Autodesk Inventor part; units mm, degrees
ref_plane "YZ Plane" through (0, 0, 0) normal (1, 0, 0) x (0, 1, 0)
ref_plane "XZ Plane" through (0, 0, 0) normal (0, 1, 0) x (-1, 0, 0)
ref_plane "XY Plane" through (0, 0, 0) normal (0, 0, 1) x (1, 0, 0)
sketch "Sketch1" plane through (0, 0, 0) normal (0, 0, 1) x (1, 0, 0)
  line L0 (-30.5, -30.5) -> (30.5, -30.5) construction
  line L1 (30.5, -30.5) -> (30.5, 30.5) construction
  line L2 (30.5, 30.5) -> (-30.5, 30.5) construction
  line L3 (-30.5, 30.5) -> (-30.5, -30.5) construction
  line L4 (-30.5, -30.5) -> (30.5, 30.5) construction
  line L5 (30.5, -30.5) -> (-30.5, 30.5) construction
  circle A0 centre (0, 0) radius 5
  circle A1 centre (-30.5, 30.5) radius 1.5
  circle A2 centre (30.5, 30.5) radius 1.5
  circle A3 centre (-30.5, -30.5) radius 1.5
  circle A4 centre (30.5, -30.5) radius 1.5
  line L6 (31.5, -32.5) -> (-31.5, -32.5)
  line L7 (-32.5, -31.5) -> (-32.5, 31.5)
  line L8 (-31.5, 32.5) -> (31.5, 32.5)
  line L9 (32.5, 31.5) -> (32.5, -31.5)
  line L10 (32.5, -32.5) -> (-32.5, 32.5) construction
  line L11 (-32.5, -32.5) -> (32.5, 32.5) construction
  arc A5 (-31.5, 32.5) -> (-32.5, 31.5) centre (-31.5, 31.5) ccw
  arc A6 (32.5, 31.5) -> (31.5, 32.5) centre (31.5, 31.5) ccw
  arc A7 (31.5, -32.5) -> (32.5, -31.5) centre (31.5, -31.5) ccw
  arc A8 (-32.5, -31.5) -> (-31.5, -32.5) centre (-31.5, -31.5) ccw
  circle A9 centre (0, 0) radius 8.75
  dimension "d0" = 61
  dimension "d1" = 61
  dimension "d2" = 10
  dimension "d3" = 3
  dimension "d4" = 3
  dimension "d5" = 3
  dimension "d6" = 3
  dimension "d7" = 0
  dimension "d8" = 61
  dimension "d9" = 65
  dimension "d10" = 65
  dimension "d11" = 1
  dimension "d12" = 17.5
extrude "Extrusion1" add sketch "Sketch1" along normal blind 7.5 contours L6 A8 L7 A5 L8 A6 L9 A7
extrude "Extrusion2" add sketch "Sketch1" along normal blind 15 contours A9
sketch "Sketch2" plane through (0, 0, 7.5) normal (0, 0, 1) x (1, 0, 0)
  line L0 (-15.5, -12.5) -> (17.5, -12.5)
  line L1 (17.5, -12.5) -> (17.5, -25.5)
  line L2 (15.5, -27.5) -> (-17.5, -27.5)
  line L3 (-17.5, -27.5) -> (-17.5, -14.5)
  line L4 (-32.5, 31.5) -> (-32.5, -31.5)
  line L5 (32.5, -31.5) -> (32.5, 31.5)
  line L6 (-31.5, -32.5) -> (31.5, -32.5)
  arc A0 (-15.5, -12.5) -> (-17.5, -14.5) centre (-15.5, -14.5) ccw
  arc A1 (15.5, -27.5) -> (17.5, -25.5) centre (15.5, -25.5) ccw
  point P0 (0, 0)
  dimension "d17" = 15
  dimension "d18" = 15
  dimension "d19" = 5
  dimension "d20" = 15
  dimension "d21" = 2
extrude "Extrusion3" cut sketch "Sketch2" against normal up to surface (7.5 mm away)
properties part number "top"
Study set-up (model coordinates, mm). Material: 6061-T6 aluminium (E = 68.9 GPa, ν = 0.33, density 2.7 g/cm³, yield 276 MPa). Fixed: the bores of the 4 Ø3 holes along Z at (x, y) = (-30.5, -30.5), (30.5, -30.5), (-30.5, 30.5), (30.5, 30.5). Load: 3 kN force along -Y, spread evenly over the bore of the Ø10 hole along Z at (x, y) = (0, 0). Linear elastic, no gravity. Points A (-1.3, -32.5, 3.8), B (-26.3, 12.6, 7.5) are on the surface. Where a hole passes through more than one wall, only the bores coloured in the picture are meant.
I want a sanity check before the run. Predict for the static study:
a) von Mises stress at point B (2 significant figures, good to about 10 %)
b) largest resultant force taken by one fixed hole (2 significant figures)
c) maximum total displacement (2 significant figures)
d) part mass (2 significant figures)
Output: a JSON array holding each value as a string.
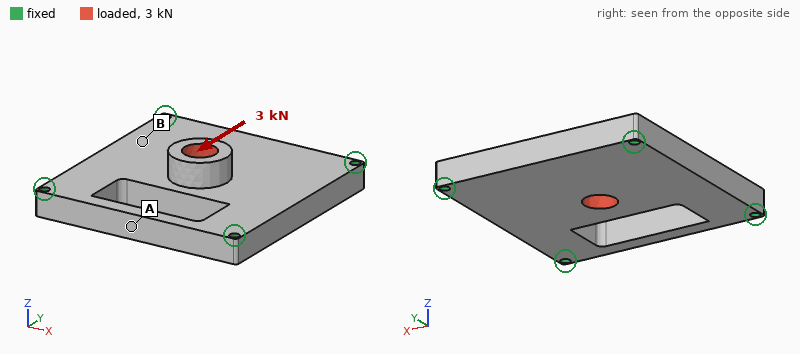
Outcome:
["10 MPa", "1.0 kN", "25 µm", "76 g"]
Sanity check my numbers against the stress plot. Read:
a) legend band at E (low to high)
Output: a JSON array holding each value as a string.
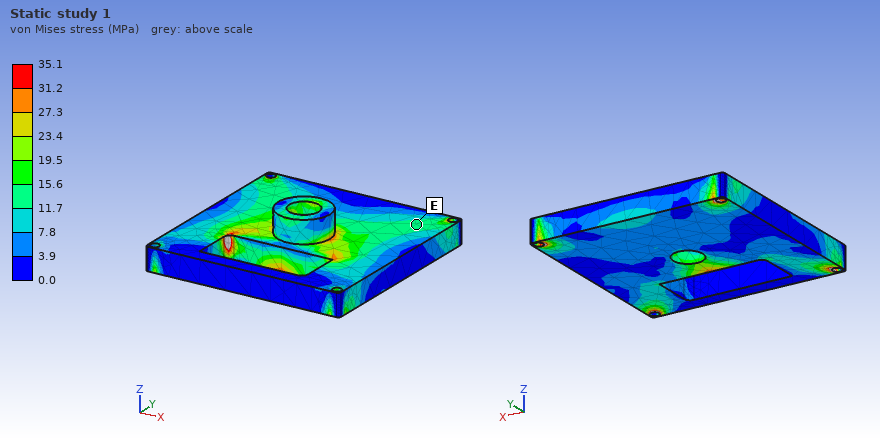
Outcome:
["11.7 to 15.6 MPa"]
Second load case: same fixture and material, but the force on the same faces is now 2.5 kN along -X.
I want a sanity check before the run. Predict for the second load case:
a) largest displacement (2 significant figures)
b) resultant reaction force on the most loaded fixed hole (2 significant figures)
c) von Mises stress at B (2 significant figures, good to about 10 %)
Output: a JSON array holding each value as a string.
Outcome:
["17 µm", "1.2 kN", "7.4 MPa"]
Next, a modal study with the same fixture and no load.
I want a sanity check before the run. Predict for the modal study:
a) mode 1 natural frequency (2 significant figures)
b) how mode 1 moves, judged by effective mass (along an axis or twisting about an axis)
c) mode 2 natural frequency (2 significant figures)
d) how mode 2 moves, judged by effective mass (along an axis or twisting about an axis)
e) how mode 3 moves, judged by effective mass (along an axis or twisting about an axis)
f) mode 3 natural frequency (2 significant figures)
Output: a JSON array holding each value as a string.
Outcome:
["5200 Hz", "along Z", "9100 Hz", "twisting about Y", "twisting about X", "10000 Hz"]
